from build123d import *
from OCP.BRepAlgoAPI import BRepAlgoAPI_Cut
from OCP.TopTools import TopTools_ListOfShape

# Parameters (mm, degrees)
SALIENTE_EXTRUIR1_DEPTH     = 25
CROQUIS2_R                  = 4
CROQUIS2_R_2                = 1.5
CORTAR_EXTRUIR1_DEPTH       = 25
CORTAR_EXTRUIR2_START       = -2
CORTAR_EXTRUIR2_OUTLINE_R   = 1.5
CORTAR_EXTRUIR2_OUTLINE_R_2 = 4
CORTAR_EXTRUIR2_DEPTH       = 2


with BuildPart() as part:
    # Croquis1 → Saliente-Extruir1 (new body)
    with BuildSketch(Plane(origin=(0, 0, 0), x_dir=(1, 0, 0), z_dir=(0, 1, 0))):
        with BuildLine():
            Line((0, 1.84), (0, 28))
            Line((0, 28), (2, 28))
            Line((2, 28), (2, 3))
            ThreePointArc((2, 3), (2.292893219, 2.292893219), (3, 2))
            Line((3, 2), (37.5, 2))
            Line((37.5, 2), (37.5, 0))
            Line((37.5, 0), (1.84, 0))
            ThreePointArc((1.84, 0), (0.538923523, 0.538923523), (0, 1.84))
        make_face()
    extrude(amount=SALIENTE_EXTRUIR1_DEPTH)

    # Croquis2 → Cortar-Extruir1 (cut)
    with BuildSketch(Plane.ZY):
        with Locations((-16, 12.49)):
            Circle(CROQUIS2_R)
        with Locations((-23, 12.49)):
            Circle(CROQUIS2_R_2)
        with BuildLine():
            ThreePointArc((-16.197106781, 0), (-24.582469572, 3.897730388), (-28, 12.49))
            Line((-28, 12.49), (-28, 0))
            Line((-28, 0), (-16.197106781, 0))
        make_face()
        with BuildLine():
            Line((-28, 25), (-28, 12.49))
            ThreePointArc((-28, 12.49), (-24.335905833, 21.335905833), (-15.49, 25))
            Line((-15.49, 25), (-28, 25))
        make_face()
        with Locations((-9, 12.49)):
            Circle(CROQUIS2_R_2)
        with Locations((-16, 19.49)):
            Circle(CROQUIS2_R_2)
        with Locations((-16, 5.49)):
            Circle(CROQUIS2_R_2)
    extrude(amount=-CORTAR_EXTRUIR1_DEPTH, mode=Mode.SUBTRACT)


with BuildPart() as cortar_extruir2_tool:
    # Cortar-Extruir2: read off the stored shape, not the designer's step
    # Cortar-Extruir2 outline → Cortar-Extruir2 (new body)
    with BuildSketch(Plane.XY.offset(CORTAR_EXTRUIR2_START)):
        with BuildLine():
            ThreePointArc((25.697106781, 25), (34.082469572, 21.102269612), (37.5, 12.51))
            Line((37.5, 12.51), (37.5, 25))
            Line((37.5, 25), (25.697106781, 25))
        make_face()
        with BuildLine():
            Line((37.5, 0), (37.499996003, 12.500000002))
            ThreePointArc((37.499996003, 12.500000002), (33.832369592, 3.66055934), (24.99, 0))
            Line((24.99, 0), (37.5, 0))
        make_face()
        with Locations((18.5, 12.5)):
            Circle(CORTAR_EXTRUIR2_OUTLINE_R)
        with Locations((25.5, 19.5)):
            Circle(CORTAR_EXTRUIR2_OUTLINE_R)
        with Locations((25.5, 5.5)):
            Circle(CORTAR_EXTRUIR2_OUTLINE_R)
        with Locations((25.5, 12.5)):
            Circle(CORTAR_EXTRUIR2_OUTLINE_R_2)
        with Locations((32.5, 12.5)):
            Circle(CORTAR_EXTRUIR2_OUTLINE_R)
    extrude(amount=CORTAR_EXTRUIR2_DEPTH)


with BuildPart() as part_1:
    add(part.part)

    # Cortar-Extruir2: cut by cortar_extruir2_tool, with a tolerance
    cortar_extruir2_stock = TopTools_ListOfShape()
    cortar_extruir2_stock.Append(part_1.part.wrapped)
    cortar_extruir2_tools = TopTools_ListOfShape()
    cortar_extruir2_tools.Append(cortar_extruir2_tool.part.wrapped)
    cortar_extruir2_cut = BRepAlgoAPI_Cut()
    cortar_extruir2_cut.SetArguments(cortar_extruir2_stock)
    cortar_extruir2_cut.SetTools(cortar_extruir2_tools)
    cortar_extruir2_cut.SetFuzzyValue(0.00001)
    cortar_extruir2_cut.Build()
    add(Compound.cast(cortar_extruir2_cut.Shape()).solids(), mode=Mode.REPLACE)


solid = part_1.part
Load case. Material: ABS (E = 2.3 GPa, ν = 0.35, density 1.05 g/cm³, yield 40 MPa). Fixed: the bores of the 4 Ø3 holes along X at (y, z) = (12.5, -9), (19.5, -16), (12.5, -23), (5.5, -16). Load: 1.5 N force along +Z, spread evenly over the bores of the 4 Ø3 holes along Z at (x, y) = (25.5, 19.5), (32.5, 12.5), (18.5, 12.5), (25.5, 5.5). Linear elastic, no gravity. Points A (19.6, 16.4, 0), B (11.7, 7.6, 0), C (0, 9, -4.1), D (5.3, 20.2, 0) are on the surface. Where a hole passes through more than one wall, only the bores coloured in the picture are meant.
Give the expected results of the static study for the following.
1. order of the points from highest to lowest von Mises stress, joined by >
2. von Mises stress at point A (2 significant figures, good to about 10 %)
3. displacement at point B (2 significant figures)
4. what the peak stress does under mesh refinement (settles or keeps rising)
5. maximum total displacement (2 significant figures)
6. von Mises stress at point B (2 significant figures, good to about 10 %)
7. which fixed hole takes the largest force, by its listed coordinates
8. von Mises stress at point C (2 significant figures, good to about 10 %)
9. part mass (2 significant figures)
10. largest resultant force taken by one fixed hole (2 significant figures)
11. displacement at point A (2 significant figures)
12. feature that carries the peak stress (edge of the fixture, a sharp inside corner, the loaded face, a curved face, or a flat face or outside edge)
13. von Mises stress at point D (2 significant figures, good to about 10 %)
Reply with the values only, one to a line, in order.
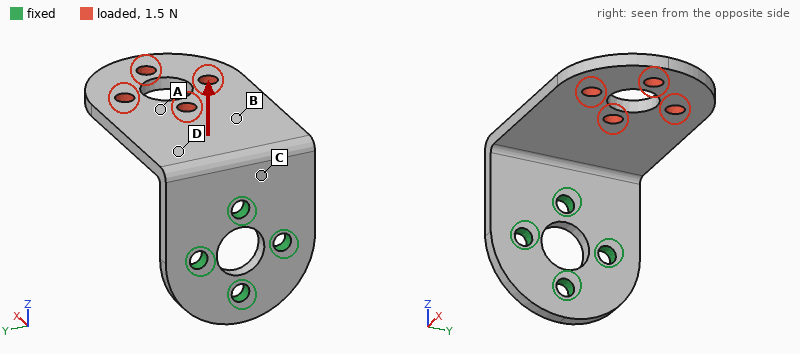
C > D > B > A
0.62 MPa
0.12 mm
keeps rising
0.56 mm
1.1 MPa
(12.5, -9)
2.1 MPa
2.7 g
2.9 N
0.24 mm
edge of the fixture
1.6 MPa
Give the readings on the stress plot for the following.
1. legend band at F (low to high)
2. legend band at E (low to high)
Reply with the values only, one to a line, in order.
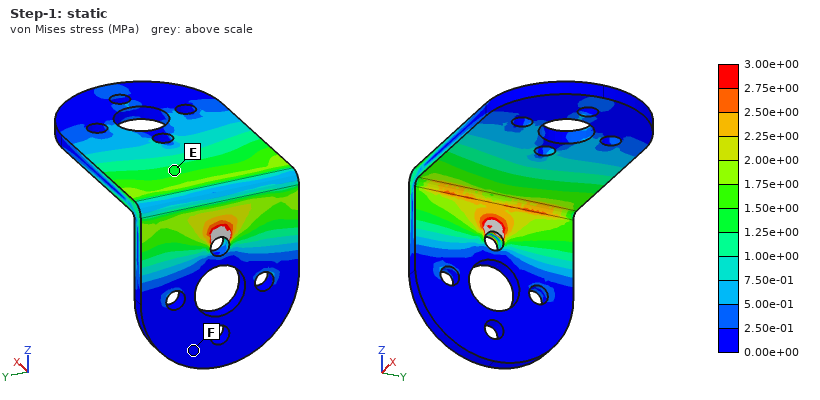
0.00e+00 to 2.50e-01 MPa
1.25e+00 to 1.50e+00 MPa
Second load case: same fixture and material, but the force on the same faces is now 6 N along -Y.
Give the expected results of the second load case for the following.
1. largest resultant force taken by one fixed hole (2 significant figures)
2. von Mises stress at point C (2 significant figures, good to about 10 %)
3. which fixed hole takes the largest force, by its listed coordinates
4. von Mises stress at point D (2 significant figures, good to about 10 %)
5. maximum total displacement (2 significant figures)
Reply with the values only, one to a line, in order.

5.8 N
3.5 MPa
(12.5, -9)
1.9 MPa
0.53 mm
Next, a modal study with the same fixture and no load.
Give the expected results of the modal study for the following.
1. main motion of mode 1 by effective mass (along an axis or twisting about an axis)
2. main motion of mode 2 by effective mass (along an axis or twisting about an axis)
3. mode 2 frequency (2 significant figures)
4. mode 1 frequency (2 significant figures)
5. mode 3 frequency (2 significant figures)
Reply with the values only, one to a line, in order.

along Z
along Y
610 Hz
340 Hz
1300 Hz
